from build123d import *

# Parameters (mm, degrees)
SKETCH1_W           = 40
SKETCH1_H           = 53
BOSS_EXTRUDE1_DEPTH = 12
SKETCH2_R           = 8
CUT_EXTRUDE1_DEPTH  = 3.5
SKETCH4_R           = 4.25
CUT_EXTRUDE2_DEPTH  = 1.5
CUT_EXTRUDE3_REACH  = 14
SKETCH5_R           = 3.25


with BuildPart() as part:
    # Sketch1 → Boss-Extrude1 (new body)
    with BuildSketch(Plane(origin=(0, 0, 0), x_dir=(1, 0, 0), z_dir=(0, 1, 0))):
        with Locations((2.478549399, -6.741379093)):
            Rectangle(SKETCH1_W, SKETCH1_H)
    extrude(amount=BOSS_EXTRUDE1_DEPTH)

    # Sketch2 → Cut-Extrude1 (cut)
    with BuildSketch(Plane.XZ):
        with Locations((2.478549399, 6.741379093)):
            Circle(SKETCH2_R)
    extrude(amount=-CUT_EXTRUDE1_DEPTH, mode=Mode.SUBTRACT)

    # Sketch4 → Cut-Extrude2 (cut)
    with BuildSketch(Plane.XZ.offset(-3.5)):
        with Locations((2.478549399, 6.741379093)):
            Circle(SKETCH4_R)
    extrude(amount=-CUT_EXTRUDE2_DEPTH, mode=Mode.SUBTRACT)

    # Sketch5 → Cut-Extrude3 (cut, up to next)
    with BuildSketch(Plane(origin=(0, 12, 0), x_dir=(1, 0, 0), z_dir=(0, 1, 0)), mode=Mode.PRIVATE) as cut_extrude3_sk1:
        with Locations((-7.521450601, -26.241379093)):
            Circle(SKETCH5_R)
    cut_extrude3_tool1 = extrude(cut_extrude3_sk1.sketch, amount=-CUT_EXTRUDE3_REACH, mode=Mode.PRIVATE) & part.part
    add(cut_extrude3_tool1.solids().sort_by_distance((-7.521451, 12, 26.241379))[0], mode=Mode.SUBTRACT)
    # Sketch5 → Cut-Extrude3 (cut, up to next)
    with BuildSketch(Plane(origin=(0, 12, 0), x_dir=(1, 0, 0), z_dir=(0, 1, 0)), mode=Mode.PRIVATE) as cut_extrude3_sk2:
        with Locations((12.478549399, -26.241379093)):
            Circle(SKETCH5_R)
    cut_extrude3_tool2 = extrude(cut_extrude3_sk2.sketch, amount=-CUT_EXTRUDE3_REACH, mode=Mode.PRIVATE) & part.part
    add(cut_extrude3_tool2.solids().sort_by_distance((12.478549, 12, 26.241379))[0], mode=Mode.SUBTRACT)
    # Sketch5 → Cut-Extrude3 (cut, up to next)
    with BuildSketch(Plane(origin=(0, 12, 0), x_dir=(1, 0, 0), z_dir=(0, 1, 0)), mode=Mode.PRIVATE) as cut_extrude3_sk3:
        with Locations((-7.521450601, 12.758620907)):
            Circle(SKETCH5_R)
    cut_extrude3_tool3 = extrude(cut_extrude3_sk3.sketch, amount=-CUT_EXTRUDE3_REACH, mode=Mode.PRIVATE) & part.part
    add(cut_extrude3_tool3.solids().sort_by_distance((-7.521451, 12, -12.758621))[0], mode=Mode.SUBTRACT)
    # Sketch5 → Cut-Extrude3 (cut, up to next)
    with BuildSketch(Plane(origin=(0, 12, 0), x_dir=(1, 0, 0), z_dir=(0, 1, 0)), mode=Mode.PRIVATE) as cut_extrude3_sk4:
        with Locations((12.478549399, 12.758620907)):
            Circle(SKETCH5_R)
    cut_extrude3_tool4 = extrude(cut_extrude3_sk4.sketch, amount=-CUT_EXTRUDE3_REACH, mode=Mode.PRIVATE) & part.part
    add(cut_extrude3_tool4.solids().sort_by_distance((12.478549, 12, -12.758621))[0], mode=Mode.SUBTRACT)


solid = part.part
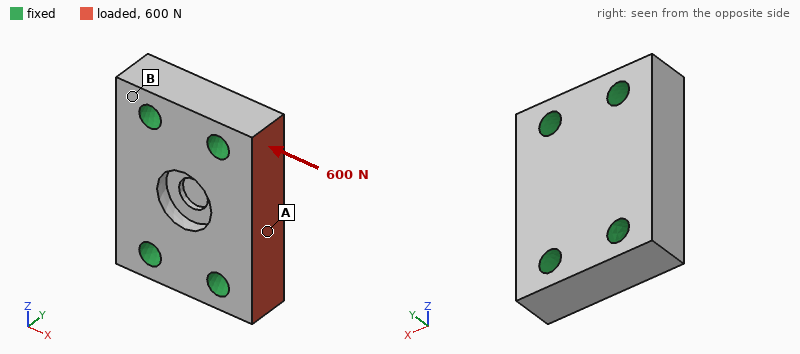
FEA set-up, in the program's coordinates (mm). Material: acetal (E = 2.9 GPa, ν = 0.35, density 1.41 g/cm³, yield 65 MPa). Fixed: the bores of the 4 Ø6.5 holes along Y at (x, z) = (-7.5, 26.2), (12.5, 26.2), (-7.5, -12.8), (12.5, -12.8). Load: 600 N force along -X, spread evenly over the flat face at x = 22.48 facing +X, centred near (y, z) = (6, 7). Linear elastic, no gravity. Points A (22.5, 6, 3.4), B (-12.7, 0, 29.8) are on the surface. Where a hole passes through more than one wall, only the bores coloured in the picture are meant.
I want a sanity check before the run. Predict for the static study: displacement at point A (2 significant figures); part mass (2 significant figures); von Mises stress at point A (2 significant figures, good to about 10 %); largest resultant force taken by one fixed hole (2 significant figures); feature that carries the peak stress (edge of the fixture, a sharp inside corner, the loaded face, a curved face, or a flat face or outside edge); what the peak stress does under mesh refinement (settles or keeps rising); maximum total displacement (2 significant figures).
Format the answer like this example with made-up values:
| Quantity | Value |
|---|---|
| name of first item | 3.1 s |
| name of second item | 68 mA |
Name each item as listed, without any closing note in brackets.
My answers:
| Quantity | Value |
|---|---|
| displacement at point A | 8.6 µm |
| part mass | 33 g |
| von Mises stress at point A | 0.99 MPa |
| largest resultant force taken by one fixed hole | 230 N |
| feature that carries the peak stress | edge of the fixture |
| what the peak stress does under mesh refinement | keeps rising |
| maximum total displacement | 9.9 µm |
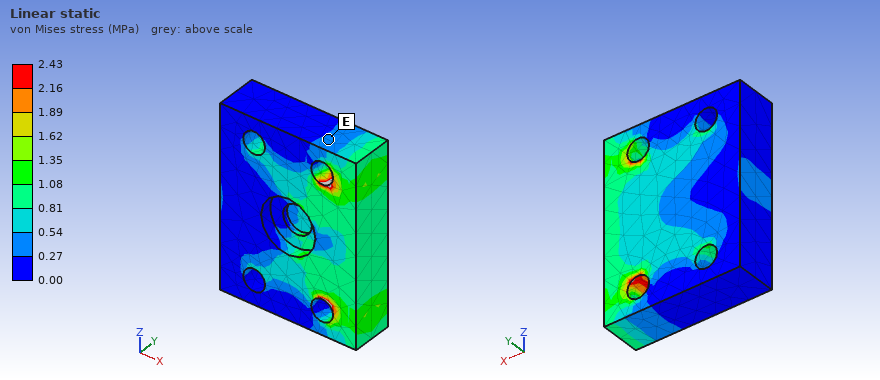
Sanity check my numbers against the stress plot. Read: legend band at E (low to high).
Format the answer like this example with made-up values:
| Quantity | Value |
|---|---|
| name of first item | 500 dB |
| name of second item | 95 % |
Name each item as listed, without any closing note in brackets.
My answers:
| Quantity | Value |
|---|---|
| legend band at E | 0.27 to 0.54 MPa |
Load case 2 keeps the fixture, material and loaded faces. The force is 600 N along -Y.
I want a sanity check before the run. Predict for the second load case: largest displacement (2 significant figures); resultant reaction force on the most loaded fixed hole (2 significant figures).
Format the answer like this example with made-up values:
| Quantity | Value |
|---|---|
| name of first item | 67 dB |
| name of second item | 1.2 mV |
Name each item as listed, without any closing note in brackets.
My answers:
| Quantity | Value |
|---|---|
| largest displacement | 50 µm |
| resultant reaction force on the most loaded fixed hole | 330 N |
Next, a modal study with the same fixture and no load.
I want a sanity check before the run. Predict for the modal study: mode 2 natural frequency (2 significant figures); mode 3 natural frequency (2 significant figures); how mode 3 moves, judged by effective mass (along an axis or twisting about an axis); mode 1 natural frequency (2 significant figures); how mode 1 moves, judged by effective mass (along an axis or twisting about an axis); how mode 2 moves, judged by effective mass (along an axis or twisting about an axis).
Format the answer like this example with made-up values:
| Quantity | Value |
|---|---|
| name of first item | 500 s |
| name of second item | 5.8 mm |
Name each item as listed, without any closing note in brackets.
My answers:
| Quantity | Value |
|---|---|
| mode 2 natural frequency | 8800 Hz |
| mode 3 natural frequency | 11 kHz |
| how mode 3 moves, judged by effective mass | along X |
| mode 1 natural frequency | 8300 Hz |
| how mode 1 moves, judged by effective mass | along Y |
| how mode 2 moves, judged by effective mass | twisting about Z |
